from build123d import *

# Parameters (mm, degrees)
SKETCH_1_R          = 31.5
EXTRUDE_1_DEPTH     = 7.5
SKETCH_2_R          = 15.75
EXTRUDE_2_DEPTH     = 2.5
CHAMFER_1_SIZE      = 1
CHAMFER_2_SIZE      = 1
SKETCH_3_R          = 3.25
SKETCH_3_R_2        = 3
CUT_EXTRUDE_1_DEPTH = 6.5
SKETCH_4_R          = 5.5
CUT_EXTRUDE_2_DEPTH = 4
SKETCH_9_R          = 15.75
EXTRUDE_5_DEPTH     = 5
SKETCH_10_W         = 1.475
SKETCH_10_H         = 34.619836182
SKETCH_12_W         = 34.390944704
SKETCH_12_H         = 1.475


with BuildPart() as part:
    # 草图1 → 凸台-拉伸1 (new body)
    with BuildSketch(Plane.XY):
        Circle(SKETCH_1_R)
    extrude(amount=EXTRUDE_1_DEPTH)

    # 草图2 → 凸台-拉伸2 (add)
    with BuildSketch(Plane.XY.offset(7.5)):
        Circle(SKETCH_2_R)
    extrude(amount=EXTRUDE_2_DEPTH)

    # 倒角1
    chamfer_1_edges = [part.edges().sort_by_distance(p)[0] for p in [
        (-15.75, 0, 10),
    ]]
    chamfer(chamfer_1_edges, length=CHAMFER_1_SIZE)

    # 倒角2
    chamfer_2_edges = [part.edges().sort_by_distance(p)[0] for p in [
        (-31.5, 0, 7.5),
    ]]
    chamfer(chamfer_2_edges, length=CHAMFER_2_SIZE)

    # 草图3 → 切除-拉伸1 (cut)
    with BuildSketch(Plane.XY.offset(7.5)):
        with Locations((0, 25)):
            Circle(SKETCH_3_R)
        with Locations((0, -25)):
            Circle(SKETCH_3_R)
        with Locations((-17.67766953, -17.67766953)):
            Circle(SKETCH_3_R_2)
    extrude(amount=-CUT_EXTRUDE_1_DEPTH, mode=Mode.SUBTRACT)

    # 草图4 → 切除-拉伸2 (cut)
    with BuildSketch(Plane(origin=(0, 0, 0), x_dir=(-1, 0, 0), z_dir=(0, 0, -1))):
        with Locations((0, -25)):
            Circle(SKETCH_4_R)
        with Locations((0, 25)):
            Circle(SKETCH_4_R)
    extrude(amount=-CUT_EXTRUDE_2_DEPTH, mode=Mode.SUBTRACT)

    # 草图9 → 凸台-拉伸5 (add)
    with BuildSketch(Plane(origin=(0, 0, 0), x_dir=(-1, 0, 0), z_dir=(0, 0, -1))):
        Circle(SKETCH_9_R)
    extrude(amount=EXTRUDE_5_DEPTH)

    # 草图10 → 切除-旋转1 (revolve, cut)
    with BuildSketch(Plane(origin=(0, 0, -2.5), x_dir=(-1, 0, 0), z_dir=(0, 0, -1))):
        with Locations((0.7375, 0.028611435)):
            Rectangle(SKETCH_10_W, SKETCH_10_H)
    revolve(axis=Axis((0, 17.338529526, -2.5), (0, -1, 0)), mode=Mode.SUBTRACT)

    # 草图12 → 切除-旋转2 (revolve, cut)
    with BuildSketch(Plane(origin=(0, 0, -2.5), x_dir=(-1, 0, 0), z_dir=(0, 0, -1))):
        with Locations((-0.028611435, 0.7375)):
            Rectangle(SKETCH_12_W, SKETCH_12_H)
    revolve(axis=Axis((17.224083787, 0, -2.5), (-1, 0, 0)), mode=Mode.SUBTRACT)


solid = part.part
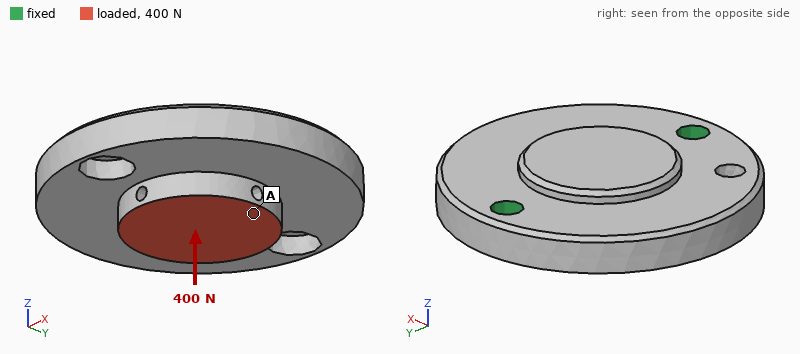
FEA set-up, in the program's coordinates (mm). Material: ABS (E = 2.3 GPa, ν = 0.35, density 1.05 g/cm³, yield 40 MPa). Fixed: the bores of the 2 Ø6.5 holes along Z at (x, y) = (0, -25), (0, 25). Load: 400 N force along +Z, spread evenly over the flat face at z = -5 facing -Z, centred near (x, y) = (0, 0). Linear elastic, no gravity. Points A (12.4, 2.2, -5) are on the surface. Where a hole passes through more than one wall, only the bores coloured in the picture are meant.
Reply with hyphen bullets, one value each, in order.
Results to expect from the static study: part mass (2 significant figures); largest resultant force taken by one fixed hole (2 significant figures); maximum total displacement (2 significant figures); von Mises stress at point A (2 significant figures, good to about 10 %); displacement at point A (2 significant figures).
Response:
- 29 g
- 230 N
- 95 µm
- 2.2 MPa
- 72 µm
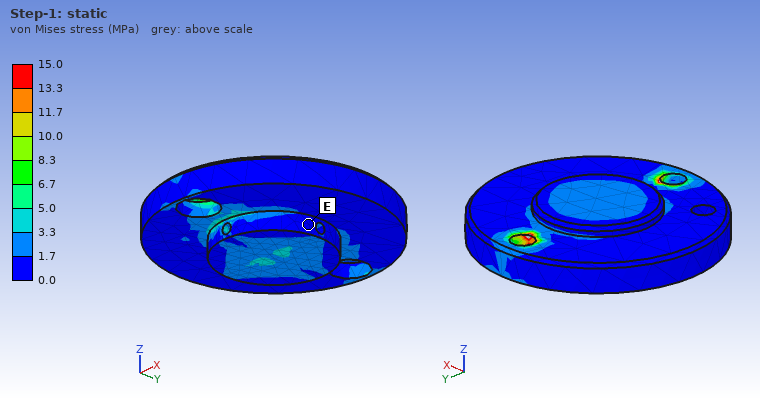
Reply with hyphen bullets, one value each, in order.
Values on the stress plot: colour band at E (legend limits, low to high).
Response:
- 0.0 to 1.7 MPa
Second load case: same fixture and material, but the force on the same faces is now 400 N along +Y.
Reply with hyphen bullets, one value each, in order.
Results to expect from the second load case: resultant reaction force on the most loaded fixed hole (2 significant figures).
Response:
- 220 N
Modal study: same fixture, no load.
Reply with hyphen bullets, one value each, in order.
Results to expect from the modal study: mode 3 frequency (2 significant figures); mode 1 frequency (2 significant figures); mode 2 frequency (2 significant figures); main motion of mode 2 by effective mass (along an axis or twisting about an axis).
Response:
- 4300 Hz
- 1000 Hz
- 2200 Hz
- along Z
